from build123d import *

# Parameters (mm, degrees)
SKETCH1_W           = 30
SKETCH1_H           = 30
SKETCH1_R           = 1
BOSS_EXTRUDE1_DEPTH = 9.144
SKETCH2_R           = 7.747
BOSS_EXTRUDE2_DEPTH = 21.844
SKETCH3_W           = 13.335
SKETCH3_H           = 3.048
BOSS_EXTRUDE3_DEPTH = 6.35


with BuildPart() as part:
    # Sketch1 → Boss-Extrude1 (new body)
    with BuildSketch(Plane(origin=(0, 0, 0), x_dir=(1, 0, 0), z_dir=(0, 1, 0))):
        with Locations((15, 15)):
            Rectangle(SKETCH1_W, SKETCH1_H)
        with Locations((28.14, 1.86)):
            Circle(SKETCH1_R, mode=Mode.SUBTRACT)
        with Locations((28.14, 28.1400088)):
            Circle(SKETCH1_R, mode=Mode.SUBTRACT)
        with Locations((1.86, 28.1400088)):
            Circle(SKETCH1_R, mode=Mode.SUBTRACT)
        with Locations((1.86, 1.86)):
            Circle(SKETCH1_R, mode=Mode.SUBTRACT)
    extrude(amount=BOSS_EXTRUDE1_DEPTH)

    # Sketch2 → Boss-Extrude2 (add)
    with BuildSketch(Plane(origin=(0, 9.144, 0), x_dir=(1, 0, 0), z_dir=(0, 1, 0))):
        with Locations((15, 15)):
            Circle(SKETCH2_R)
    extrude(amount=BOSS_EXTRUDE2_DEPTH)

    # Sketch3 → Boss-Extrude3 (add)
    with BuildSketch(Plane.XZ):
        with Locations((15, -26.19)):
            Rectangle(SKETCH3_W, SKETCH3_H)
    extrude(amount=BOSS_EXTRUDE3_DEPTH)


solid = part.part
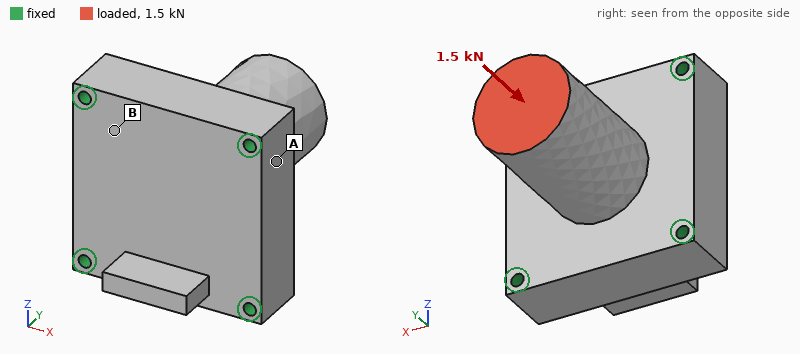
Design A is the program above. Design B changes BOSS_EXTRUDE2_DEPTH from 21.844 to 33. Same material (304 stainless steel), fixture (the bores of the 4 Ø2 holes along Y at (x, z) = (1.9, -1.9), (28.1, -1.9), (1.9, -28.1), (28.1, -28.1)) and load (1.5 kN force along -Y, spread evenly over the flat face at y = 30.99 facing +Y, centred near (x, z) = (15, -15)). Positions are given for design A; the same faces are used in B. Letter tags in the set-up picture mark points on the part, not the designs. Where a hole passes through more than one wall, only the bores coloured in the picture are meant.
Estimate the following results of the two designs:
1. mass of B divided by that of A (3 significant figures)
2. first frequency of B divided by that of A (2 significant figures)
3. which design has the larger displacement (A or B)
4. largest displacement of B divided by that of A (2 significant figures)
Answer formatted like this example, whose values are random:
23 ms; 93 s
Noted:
1.17; 0.54; B; 1.2
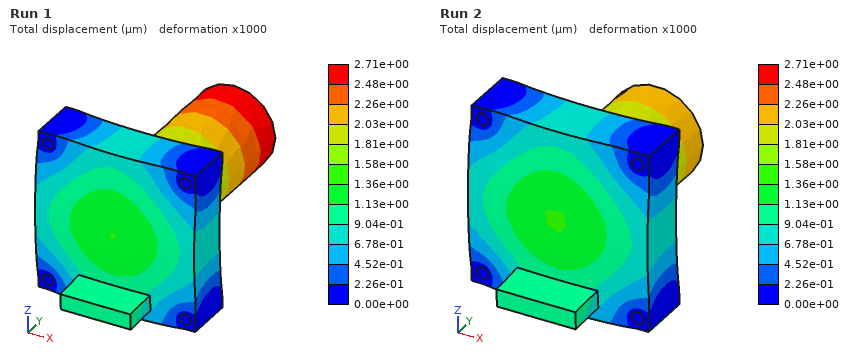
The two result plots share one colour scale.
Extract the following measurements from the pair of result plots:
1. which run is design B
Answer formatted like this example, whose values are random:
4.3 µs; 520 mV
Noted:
Run 1
